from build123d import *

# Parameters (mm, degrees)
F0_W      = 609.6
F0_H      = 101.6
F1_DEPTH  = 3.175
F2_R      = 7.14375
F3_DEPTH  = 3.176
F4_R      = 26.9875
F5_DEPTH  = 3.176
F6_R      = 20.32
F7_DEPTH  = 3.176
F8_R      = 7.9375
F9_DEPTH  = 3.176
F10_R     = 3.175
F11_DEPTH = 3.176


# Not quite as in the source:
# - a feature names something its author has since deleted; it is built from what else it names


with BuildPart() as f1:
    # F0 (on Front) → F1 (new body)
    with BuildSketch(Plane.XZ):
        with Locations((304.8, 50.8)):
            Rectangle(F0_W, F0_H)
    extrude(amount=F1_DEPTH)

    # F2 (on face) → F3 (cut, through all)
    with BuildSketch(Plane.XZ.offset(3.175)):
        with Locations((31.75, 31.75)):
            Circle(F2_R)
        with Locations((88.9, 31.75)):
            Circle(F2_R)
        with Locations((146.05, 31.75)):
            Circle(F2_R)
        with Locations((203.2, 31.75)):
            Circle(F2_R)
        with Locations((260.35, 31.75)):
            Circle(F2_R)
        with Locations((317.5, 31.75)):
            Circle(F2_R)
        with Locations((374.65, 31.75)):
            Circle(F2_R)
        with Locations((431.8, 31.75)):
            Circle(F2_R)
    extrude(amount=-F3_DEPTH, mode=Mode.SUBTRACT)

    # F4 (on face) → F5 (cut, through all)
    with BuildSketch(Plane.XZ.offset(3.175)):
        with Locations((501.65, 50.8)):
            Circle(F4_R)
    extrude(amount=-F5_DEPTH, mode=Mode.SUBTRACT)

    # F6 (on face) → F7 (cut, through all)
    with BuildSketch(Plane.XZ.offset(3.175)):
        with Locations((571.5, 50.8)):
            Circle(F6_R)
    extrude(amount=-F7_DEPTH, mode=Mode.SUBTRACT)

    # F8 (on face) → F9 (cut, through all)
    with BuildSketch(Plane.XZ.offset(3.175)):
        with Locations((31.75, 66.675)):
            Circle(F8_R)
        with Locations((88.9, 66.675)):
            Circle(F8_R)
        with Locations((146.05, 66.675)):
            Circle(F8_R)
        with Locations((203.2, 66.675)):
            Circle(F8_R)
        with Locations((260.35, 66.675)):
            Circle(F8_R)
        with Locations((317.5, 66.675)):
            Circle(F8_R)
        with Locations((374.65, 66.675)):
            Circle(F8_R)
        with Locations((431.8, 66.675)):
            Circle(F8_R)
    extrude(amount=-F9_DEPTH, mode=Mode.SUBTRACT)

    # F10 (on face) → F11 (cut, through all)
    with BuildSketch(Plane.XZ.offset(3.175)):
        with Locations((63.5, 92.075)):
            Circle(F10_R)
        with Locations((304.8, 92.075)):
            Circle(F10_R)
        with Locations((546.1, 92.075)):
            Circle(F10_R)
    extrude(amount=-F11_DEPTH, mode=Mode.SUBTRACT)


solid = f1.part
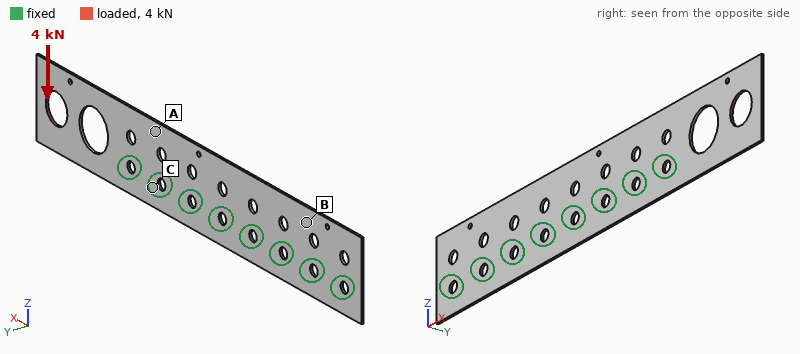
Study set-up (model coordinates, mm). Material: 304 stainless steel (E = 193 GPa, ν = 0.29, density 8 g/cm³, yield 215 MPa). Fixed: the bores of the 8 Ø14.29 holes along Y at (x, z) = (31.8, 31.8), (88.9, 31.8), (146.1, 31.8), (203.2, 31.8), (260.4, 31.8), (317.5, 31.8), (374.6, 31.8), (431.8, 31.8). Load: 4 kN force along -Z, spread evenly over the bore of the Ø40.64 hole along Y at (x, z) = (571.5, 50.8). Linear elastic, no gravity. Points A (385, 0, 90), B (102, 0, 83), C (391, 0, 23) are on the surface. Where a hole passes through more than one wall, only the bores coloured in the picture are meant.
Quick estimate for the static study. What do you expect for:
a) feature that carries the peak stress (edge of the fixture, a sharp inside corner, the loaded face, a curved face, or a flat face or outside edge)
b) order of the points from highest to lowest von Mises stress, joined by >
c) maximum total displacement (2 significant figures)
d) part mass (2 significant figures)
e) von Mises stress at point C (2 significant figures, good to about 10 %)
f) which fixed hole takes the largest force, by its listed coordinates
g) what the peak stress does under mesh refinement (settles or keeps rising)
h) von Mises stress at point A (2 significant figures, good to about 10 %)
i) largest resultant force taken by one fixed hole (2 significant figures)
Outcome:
edge of the fixture
A > C > B
0.31 mm
1.4 kg
32 MPa
(431.8, 31.8)
keeps rising
50 MPa
9.2 kN
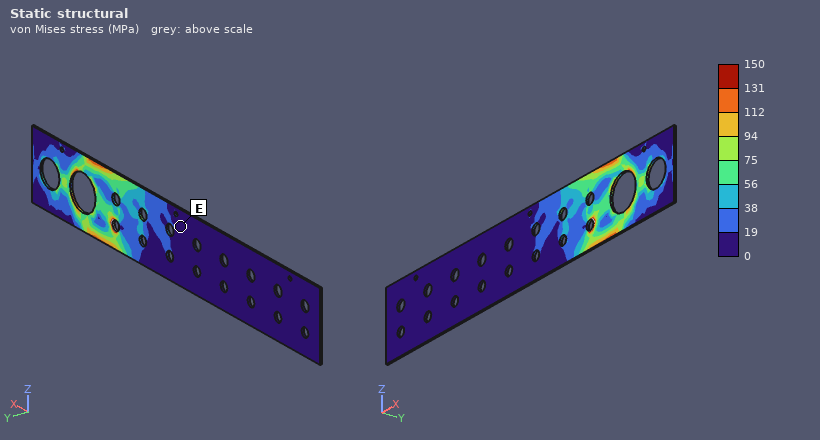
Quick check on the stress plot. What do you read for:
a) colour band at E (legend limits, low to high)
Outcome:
0 to 19 MPa
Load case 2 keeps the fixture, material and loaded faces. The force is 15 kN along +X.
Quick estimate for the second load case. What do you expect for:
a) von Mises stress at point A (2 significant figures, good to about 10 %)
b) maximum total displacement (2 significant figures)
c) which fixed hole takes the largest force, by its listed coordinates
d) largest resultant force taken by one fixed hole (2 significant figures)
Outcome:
36 MPa
97 µm
(431.8, 31.8)
9.7 kN
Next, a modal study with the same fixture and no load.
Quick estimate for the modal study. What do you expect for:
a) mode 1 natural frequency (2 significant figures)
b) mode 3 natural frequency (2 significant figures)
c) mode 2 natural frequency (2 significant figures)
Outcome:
77 Hz
450 Hz
240 Hz
